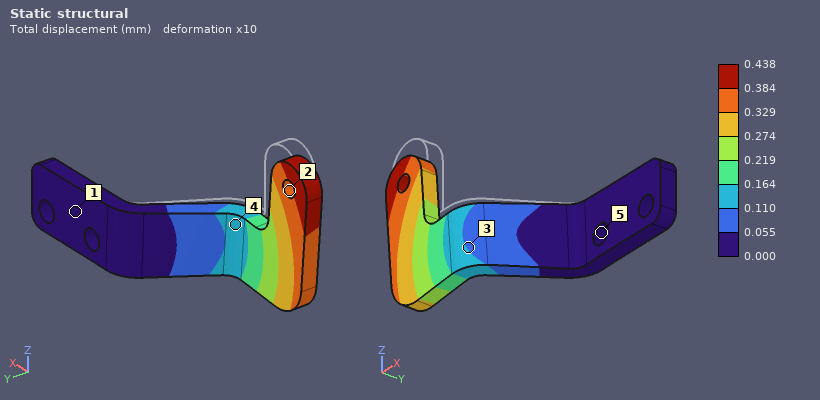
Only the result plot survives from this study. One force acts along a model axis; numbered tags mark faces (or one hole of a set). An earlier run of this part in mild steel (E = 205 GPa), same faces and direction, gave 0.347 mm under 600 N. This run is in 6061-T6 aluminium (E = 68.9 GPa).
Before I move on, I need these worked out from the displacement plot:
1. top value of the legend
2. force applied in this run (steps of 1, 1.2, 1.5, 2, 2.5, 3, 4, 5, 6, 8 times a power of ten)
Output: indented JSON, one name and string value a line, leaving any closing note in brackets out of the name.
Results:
{
  "top value of the legend": "0.438 mm",
  "force applied in this run": "250 N"
}
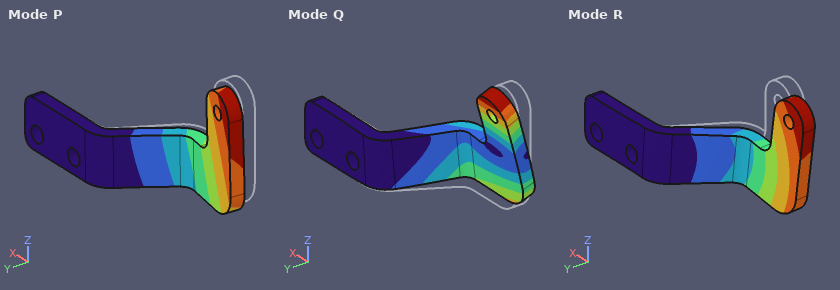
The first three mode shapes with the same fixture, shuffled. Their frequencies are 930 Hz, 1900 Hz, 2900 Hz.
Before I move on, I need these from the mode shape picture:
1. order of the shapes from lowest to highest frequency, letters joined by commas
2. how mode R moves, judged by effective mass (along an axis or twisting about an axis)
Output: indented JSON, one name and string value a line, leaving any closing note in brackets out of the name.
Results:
{
  "order of the shapes from lowest to highest frequency, letters joined by commas": "P, R, Q",
  "how mode R moves, judged by effective mass": "along Z"
}
